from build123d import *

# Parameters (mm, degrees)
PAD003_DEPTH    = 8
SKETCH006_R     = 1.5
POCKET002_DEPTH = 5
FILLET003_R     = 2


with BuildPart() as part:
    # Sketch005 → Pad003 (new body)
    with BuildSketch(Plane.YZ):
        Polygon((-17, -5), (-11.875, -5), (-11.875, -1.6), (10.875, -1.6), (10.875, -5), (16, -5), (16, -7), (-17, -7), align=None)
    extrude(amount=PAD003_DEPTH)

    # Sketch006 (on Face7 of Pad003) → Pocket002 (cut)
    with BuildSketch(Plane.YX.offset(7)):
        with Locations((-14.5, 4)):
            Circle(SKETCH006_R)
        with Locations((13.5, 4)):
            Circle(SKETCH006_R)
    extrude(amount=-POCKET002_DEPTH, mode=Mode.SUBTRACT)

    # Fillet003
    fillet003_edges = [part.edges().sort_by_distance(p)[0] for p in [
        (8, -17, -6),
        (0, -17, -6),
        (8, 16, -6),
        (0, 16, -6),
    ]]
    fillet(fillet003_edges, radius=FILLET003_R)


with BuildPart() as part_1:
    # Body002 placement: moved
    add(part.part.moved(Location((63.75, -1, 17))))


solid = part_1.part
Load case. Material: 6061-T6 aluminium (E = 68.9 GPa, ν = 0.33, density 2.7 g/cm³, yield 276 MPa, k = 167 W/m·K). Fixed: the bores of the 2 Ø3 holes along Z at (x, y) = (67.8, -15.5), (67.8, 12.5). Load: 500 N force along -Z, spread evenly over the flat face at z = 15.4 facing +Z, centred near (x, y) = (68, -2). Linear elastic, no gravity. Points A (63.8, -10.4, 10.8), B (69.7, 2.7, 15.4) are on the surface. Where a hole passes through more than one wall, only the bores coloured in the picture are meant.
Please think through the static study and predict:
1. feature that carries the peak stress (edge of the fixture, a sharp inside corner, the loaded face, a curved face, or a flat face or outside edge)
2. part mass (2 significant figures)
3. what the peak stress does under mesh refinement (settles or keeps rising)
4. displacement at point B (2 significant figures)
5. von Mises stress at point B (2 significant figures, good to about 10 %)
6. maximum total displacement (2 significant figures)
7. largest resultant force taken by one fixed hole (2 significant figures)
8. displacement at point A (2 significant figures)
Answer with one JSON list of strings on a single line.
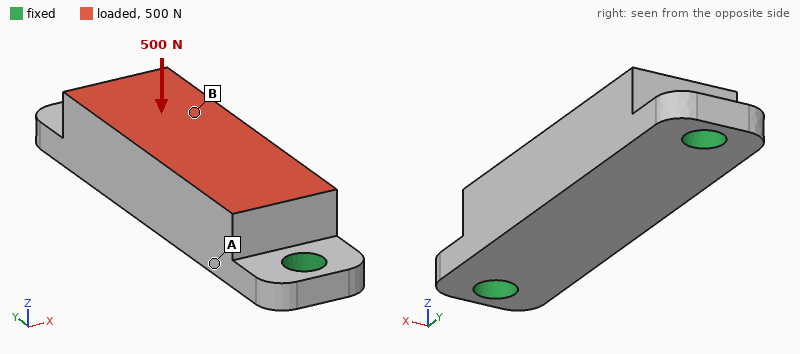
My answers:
["edge of the fixture", "3.0 g", "keeps rising", "10 µm", "26 MPa", "12 µm", "350 N", "6.2 µm"]
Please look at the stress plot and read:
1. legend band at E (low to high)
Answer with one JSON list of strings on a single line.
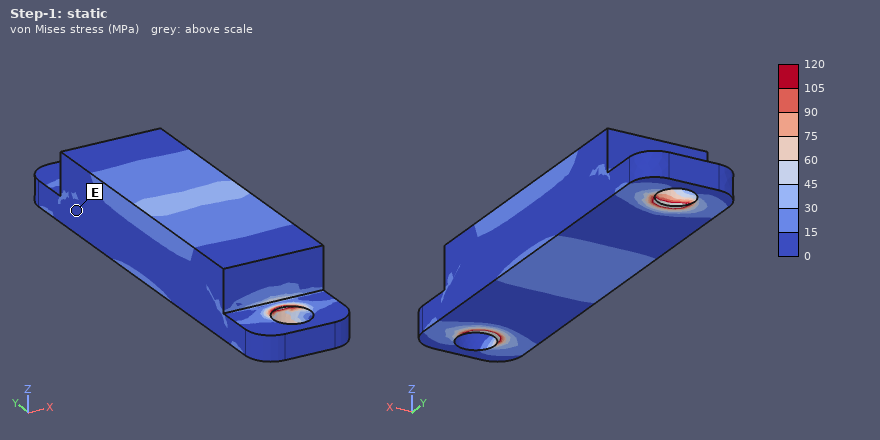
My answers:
["0 to 15 MPa"]
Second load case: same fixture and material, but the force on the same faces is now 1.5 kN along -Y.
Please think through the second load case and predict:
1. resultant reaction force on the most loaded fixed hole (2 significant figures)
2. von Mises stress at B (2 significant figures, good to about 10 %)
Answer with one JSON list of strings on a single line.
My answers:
["800 N", "15 MPa"]
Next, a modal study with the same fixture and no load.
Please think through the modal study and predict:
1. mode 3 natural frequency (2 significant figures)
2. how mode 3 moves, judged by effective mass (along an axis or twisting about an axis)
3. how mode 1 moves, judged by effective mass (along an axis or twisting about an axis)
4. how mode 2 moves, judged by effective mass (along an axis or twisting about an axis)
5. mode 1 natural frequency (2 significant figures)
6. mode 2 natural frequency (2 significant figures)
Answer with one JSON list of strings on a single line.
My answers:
["33 kHz", "along X", "along X", "along Z", "20 kHz", "22 kHz"]
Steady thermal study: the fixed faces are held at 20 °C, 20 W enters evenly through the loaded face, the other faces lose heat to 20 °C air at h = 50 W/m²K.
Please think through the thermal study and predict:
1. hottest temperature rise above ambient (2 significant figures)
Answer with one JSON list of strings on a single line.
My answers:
["20 K"]
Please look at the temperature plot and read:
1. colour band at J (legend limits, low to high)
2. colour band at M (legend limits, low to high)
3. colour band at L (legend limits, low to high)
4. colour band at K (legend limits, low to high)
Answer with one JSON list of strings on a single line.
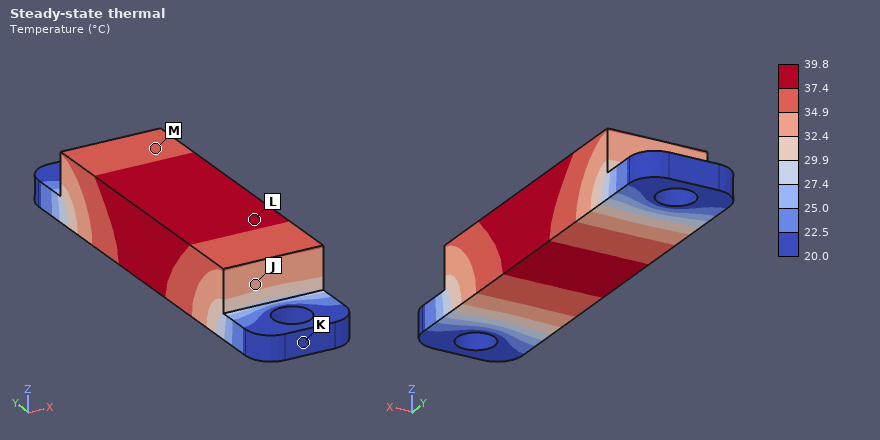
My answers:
["32.4 to 34.9 °C", "34.9 to 37.4 °C", "37.4 to 39.8 °C", "20.0 to 22.5 °C"]
